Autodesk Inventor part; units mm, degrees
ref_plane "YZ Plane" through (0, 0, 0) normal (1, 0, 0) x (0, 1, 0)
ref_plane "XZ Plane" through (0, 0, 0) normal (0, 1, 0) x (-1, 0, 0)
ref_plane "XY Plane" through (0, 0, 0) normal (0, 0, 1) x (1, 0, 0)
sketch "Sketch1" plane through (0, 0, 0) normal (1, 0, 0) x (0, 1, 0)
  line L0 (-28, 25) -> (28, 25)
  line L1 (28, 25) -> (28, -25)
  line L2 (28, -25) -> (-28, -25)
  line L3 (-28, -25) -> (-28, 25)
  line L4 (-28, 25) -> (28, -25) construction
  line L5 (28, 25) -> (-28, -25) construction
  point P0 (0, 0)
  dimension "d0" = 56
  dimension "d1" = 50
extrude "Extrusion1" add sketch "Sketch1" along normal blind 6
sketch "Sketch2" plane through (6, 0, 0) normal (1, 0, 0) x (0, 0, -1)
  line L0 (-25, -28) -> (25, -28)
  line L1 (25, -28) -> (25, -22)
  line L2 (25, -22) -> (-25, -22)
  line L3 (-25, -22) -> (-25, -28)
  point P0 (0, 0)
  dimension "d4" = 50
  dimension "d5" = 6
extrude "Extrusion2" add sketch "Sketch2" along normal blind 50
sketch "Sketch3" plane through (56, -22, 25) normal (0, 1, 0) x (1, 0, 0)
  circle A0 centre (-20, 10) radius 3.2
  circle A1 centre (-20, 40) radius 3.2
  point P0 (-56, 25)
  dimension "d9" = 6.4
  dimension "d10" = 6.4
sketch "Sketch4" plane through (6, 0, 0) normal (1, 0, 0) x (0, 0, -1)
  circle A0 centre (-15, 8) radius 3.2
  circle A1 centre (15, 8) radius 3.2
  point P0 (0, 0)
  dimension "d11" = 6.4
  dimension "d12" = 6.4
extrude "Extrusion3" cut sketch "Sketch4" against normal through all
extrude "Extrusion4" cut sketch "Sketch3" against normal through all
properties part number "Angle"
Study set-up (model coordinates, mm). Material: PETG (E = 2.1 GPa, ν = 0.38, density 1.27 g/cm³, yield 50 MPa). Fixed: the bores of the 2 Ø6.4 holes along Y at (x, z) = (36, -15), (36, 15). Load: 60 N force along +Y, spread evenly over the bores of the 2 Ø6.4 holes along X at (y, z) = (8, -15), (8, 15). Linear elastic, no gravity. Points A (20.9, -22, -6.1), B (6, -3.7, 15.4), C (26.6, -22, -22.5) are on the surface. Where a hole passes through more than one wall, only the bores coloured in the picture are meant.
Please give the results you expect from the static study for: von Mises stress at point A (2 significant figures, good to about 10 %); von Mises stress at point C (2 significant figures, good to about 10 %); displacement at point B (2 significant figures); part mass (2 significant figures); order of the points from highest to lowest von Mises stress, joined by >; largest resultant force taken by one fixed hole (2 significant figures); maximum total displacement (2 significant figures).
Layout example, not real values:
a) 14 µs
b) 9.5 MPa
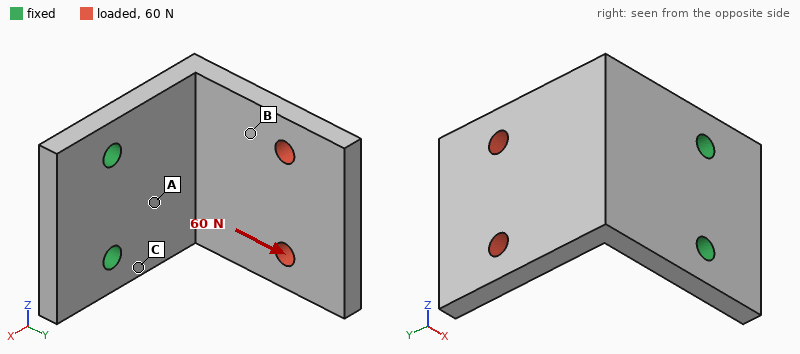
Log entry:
a) 3.1 MPa
b) 4.6 MPa
c) 0.45 mm
d) 39 g
e) C > A > B
f) 30 N
g) 0.91 mm
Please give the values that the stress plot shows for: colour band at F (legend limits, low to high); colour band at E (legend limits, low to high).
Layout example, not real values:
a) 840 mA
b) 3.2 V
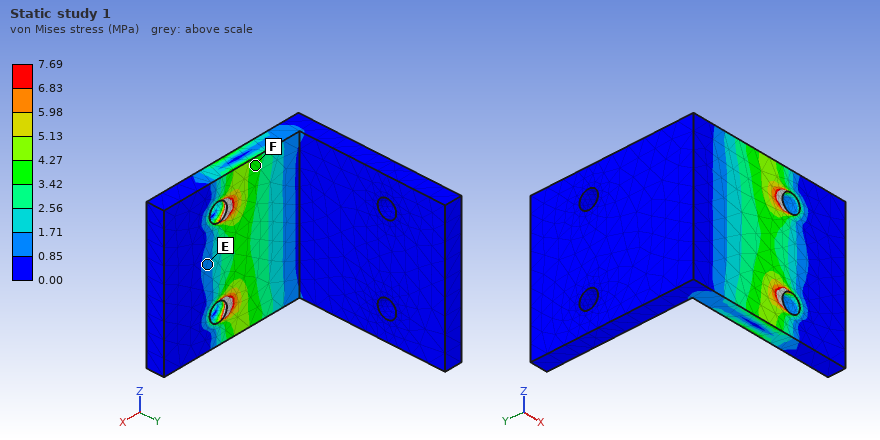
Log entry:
a) 3.42 to 4.27 MPa
b) 0.85 to 1.71 MPa
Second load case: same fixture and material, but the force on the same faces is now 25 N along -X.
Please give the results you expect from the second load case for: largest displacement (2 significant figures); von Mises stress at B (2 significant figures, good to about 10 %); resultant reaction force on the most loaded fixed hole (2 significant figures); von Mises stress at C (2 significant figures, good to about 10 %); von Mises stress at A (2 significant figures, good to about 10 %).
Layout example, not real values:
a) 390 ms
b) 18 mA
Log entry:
a) 0.96 mm
b) 0.92 MPa
c) 13 N
d) 2.7 MPa
e) 2.5 MPa
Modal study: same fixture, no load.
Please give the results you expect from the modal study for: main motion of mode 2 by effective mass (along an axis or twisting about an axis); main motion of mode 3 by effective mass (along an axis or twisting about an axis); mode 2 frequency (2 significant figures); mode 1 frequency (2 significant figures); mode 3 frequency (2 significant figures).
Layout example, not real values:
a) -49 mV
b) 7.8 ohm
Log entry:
a) along Z
b) along Y
c) 420 Hz
d) 230 Hz
e) 700 Hz
